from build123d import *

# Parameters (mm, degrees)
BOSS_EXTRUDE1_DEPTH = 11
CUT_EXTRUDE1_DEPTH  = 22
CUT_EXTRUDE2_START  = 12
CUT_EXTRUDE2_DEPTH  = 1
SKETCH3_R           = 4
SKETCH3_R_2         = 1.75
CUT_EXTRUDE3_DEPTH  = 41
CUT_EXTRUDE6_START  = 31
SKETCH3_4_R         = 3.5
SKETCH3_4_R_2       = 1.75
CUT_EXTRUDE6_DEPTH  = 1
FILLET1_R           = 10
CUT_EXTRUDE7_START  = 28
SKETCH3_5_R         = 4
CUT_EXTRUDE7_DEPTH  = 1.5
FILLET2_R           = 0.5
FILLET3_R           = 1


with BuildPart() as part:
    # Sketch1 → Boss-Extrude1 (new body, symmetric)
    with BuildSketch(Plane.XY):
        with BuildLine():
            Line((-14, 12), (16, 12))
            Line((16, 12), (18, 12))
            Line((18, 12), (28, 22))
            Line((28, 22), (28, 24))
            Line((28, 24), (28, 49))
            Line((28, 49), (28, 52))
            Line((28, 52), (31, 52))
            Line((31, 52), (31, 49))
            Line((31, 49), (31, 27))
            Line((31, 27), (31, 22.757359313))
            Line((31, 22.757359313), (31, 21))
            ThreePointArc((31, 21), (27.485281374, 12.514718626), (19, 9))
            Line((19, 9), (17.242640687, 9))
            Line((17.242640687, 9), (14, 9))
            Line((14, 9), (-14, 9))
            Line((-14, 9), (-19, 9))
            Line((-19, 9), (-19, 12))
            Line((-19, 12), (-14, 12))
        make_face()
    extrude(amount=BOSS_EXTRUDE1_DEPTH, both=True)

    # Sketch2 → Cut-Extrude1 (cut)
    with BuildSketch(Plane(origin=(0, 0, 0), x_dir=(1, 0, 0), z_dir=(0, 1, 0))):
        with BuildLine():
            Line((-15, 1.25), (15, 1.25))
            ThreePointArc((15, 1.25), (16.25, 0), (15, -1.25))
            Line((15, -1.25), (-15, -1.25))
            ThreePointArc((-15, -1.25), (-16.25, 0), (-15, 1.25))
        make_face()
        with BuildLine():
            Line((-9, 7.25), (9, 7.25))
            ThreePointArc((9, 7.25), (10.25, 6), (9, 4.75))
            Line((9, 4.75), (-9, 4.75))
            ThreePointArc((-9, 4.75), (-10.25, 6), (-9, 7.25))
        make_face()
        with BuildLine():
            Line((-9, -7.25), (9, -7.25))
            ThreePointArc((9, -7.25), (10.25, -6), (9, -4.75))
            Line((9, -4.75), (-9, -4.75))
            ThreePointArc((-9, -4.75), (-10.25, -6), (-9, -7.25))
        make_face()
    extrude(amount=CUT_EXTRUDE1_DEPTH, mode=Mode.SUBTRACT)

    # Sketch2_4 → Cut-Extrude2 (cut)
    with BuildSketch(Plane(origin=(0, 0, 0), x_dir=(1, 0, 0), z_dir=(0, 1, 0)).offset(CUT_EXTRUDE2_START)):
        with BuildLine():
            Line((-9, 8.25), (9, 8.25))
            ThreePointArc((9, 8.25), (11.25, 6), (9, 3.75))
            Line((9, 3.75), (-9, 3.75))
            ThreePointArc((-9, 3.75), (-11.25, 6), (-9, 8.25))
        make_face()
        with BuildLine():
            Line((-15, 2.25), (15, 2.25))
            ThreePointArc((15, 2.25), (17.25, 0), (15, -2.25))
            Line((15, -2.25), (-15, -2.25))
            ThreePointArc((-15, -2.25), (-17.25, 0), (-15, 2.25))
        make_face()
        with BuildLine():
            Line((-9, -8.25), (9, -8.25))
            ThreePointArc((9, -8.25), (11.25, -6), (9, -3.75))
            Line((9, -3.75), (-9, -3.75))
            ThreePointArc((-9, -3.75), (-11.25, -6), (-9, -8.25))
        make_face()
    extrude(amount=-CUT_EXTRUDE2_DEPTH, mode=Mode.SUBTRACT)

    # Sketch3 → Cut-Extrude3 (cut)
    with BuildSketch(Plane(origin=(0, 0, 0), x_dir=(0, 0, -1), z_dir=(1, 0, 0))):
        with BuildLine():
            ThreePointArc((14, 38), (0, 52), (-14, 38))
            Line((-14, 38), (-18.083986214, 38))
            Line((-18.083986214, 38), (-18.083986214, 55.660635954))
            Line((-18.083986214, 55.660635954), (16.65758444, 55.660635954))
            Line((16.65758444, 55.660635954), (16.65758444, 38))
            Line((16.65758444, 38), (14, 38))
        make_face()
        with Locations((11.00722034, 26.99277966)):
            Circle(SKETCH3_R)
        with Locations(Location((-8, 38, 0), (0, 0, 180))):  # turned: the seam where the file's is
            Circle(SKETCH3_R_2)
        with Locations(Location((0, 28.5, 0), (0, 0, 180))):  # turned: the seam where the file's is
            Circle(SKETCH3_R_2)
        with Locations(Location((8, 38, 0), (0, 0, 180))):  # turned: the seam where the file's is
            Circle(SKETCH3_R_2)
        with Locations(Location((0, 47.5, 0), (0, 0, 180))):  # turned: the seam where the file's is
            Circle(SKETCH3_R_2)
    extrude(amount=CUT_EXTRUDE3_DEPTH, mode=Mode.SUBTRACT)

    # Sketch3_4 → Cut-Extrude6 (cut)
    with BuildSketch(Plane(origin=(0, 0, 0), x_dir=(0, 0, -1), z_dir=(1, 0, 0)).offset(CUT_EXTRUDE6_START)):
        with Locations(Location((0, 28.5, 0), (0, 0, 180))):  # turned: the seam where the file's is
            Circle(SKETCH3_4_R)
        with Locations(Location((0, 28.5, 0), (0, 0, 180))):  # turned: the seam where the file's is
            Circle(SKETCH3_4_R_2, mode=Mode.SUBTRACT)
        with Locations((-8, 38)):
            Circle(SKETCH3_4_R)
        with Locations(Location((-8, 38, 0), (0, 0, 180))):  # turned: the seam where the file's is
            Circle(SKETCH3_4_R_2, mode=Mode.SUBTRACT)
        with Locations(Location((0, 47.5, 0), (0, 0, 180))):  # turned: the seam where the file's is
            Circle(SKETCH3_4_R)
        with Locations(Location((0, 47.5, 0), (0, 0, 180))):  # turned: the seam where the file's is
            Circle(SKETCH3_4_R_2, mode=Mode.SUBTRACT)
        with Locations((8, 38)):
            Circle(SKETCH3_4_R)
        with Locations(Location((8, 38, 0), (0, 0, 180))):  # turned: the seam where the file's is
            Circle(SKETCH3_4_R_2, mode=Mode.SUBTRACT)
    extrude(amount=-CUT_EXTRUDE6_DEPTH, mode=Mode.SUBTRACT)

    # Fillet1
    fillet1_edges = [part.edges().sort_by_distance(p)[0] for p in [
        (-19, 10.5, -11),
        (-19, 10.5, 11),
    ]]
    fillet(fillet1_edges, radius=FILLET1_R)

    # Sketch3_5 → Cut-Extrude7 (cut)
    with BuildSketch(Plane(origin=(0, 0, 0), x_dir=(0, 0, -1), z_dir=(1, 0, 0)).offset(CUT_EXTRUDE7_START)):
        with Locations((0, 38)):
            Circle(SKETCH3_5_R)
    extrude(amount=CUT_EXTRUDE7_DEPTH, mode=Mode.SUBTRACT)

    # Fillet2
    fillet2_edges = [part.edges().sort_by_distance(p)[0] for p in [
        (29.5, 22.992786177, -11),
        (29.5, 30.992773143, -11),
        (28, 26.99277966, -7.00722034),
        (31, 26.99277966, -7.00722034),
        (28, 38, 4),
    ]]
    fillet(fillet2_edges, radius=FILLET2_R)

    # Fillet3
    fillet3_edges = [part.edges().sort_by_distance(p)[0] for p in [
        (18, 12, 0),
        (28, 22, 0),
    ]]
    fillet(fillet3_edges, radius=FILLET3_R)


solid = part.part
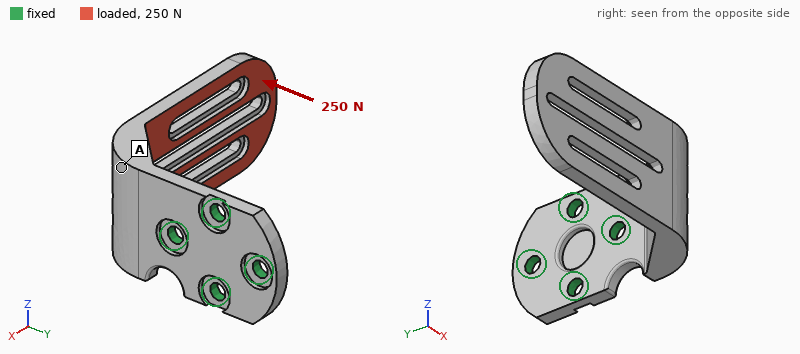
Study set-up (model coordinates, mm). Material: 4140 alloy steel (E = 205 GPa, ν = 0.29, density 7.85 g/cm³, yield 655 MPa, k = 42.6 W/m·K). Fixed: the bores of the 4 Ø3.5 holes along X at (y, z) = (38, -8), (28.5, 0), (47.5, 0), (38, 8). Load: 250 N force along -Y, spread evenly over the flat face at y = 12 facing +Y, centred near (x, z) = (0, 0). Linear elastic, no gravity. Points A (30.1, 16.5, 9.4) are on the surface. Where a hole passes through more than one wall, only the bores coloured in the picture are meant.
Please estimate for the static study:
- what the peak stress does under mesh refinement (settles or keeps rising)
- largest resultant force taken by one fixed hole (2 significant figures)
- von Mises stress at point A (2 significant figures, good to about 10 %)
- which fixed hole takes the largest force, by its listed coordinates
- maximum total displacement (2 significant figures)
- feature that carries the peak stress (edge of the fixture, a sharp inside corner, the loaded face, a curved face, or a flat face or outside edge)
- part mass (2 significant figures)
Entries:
keeps rising
870 N
67 MPa
(28.5, 0)
0.71 mm
edge of the fixture
40 g
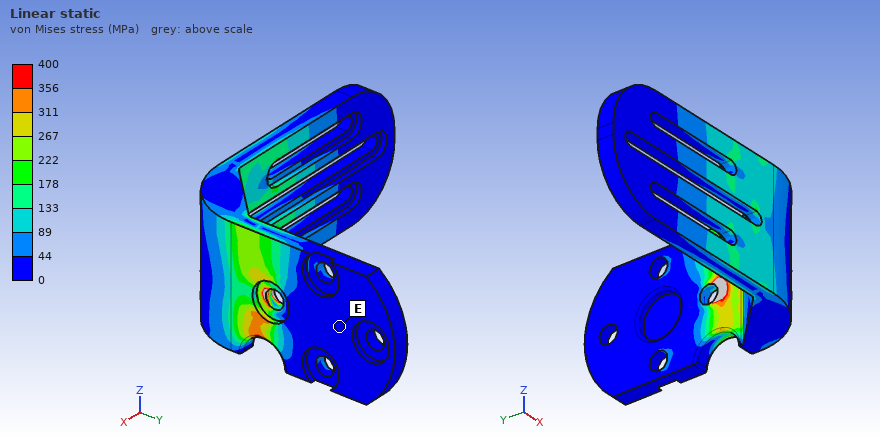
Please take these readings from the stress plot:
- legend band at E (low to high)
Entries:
0 to 44 MPa
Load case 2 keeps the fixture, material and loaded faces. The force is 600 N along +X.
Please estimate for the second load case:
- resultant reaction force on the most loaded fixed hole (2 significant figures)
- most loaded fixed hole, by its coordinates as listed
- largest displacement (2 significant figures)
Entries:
1.3 kN
(28.5, 0)
0.40 mm
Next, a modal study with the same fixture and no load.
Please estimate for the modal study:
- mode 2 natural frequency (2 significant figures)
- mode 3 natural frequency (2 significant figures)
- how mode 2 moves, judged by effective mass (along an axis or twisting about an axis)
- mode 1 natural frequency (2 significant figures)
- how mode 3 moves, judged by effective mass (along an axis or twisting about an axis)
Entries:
1600 Hz
3100 Hz
along Z
980 Hz
along X
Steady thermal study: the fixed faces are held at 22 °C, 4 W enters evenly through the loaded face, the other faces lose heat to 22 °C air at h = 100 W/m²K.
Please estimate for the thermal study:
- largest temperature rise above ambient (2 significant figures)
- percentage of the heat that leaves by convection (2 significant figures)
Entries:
21 K
76 %
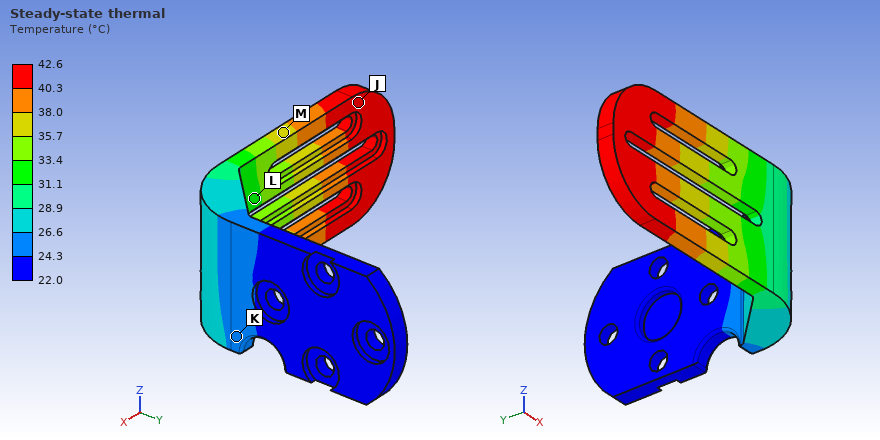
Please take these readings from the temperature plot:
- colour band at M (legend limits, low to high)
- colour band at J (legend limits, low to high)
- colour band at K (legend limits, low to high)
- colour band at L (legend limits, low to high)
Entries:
35.7 to 38.0 °C
40.3 to 42.6 °C
24.3 to 26.6 °C
31.1 to 33.4 °C
